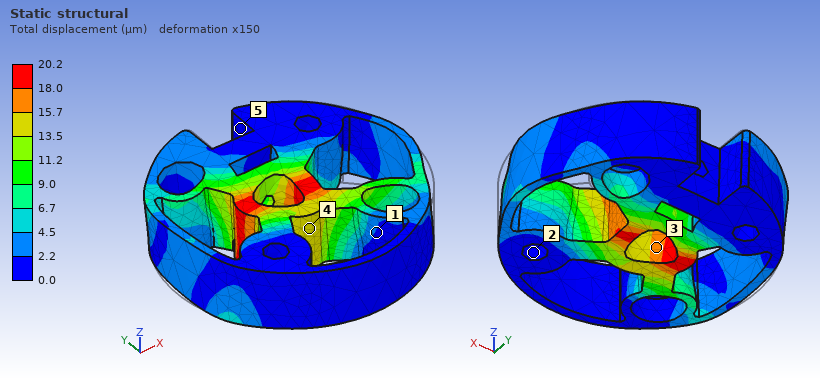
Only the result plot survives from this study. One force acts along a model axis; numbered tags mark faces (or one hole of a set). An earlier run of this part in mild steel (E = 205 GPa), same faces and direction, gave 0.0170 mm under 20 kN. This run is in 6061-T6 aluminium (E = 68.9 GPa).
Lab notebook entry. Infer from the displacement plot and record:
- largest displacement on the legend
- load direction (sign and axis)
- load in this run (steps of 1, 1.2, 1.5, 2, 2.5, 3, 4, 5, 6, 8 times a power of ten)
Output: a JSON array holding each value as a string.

["20.2 µm", "-X", "8 kN"]
